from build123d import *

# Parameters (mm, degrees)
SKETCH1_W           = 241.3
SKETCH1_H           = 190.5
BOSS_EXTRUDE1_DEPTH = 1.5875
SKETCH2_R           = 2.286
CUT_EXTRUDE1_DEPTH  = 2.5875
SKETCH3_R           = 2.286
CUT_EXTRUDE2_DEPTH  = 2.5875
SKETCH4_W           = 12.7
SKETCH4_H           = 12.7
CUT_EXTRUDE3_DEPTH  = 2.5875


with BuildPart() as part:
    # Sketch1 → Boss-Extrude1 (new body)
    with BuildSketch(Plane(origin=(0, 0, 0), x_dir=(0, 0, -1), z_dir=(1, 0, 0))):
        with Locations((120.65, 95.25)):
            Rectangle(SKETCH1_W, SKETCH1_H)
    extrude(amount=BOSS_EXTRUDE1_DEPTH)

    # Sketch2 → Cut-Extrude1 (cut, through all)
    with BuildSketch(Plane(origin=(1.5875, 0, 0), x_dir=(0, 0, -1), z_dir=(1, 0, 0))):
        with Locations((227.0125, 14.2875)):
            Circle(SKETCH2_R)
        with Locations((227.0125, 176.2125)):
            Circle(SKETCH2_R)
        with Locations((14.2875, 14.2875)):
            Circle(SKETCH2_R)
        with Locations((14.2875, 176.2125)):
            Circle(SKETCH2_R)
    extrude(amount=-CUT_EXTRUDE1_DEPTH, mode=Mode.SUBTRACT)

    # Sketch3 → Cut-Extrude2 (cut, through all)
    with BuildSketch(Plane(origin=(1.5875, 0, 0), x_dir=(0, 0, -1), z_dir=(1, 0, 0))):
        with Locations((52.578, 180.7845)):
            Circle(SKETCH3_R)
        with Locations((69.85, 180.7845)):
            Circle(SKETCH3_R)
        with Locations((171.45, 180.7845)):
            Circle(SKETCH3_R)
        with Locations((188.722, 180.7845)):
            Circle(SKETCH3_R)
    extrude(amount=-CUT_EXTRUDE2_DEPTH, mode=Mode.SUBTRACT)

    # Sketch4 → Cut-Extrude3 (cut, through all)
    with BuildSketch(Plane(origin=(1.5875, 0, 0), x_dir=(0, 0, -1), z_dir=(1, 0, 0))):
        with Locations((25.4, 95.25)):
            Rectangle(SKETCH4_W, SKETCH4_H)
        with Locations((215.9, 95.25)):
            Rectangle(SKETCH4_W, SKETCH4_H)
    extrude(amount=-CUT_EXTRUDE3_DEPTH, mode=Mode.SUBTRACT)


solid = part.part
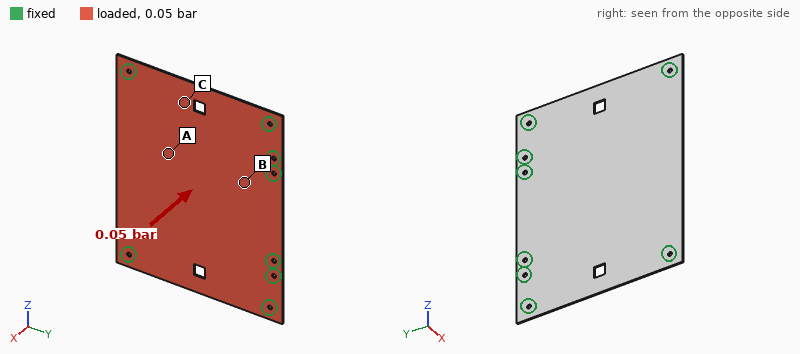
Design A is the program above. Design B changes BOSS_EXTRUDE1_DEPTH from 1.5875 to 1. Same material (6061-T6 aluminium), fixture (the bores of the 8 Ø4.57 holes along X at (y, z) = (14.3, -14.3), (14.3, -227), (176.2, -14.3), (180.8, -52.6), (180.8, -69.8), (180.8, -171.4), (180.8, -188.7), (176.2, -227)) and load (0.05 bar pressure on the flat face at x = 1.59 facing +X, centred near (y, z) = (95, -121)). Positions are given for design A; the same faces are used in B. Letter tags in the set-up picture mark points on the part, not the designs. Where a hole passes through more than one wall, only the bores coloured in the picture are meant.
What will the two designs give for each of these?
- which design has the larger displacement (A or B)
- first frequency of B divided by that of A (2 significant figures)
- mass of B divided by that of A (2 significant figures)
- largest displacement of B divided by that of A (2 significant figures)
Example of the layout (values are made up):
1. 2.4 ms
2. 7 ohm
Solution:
1. B
2. 0.63
3. 0.63
4. 4.0
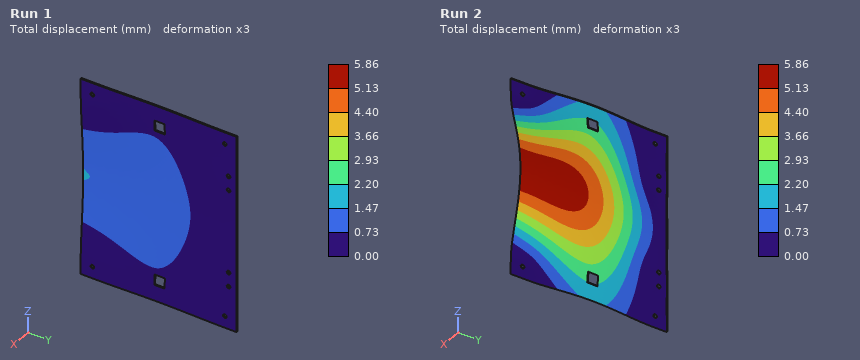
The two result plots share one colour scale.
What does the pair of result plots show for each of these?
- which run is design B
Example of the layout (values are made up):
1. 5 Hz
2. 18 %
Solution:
1. Run 2
